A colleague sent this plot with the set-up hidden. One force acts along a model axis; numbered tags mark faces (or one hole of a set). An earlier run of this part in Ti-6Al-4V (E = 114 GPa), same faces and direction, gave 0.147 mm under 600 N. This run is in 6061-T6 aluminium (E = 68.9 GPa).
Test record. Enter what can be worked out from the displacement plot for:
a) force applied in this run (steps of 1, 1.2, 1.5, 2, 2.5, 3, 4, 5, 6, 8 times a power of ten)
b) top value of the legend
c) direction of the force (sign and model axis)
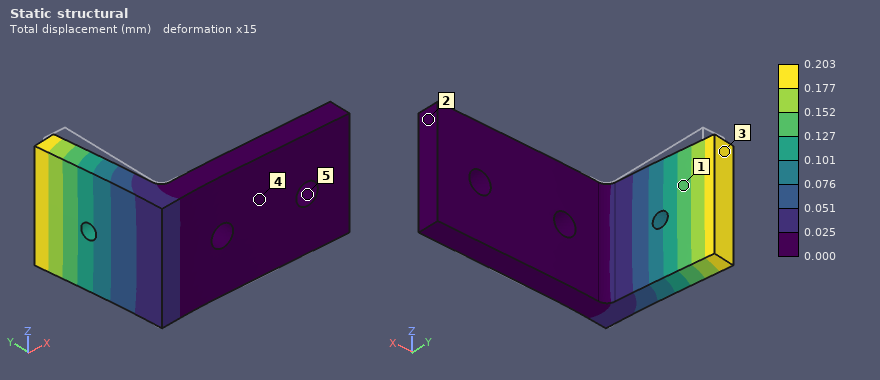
500 N
0.203 mm
-X
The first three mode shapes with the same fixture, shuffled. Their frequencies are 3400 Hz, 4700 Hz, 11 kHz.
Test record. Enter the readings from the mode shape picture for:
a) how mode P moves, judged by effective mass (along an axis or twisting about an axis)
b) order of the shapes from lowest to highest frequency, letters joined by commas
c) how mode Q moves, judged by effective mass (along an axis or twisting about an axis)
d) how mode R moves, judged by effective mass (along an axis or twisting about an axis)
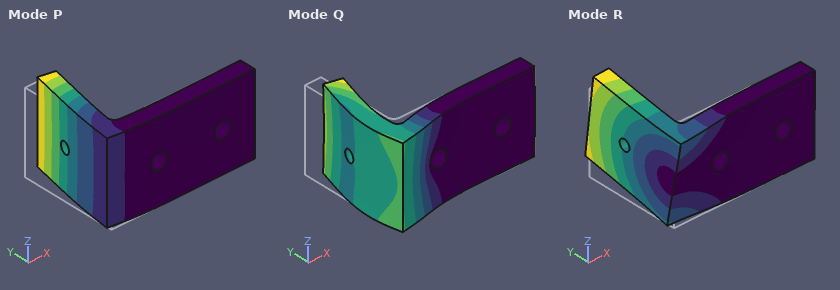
along X
P, R, Q
along Y
along Z
